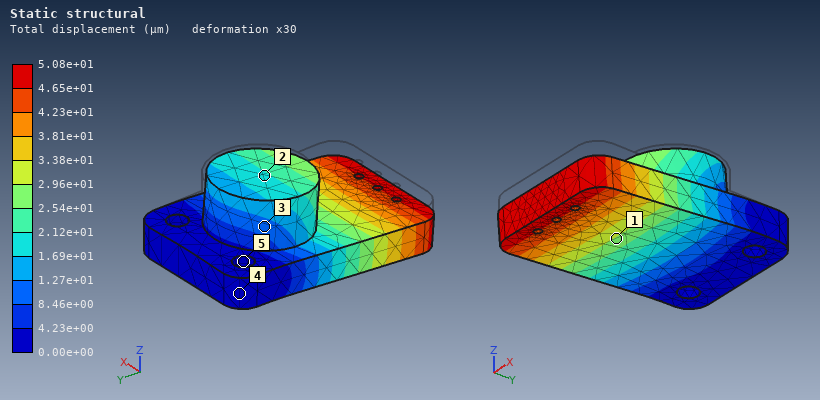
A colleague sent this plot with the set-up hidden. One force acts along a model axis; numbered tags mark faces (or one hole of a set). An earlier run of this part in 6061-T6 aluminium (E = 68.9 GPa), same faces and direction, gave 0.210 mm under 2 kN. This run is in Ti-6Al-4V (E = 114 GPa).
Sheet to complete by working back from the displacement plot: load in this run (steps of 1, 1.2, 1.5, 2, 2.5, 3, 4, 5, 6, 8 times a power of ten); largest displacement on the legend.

800 N
5.08e+01 µm
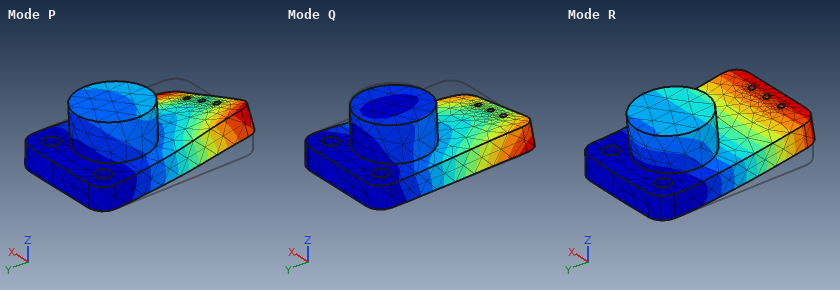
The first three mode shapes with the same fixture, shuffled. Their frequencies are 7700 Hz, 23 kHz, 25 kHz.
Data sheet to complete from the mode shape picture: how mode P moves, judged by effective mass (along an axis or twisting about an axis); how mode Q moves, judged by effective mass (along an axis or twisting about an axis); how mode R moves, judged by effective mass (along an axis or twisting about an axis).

along X
along X
along Z
